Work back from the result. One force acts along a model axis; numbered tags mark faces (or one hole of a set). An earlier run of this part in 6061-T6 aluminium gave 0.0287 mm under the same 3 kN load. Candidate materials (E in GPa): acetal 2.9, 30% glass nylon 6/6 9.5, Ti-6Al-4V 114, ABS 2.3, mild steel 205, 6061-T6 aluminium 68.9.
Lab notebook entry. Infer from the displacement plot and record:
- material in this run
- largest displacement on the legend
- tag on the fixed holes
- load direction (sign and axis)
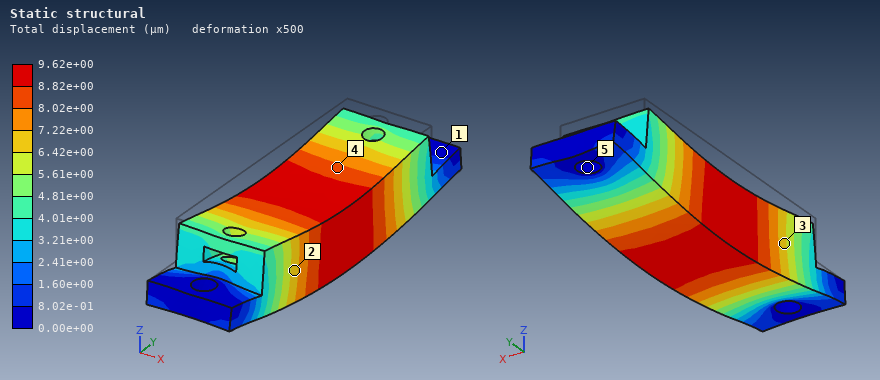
mild steel
9.62e+00 µm
5
-Z
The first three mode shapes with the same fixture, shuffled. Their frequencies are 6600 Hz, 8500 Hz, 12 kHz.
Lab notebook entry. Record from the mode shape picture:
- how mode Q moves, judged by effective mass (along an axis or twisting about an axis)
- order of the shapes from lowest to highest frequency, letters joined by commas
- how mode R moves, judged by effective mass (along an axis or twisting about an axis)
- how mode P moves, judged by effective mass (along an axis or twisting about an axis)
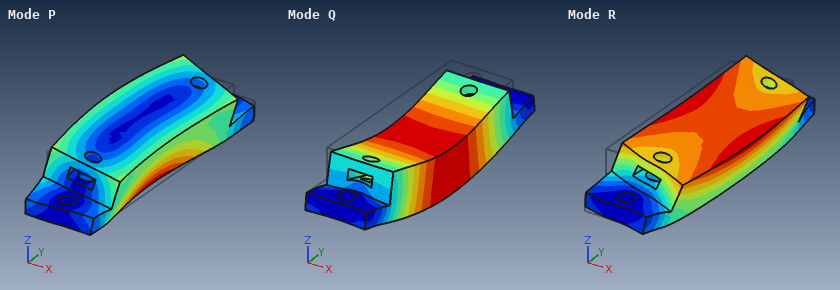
along Z
R, Q, P
along X
along X
